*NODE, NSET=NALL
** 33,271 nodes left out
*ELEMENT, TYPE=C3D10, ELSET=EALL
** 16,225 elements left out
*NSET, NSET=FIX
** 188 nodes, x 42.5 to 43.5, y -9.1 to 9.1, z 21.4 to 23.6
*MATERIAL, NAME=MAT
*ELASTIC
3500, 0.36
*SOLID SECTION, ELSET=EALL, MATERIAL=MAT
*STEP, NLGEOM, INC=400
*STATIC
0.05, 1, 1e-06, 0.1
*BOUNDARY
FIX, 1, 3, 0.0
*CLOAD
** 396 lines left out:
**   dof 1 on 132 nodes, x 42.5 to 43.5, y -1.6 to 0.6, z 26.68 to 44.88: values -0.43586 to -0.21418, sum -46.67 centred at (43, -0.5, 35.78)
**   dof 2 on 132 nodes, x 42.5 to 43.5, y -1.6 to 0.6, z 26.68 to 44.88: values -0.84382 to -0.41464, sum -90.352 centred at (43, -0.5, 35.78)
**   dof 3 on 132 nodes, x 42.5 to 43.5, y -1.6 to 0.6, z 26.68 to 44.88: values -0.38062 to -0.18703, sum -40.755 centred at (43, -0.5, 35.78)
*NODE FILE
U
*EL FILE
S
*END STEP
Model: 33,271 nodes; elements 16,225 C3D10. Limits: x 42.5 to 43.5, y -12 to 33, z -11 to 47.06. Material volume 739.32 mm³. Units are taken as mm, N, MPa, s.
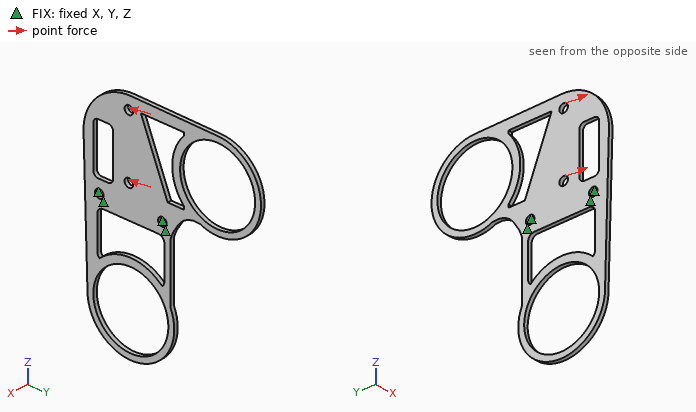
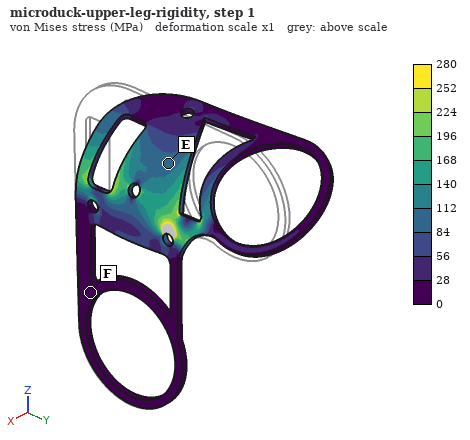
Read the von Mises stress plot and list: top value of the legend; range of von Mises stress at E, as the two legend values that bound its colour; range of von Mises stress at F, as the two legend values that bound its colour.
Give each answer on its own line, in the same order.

280 MPa
84 to 112 MPa
0 to 28 MPa
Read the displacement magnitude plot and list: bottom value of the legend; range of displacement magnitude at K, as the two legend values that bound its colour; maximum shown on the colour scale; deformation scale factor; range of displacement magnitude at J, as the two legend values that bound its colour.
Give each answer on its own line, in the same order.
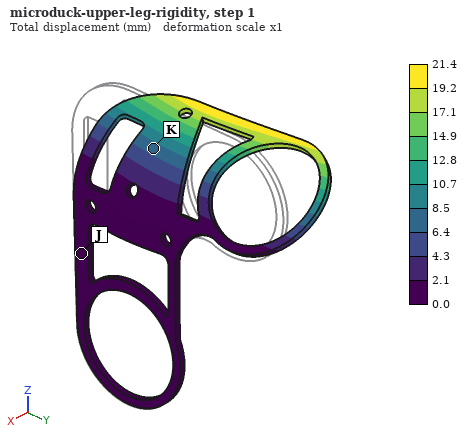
0.0 mm
6.4 to 8.5 mm
21.4 mm
1
0.0 to 2.1 mm
